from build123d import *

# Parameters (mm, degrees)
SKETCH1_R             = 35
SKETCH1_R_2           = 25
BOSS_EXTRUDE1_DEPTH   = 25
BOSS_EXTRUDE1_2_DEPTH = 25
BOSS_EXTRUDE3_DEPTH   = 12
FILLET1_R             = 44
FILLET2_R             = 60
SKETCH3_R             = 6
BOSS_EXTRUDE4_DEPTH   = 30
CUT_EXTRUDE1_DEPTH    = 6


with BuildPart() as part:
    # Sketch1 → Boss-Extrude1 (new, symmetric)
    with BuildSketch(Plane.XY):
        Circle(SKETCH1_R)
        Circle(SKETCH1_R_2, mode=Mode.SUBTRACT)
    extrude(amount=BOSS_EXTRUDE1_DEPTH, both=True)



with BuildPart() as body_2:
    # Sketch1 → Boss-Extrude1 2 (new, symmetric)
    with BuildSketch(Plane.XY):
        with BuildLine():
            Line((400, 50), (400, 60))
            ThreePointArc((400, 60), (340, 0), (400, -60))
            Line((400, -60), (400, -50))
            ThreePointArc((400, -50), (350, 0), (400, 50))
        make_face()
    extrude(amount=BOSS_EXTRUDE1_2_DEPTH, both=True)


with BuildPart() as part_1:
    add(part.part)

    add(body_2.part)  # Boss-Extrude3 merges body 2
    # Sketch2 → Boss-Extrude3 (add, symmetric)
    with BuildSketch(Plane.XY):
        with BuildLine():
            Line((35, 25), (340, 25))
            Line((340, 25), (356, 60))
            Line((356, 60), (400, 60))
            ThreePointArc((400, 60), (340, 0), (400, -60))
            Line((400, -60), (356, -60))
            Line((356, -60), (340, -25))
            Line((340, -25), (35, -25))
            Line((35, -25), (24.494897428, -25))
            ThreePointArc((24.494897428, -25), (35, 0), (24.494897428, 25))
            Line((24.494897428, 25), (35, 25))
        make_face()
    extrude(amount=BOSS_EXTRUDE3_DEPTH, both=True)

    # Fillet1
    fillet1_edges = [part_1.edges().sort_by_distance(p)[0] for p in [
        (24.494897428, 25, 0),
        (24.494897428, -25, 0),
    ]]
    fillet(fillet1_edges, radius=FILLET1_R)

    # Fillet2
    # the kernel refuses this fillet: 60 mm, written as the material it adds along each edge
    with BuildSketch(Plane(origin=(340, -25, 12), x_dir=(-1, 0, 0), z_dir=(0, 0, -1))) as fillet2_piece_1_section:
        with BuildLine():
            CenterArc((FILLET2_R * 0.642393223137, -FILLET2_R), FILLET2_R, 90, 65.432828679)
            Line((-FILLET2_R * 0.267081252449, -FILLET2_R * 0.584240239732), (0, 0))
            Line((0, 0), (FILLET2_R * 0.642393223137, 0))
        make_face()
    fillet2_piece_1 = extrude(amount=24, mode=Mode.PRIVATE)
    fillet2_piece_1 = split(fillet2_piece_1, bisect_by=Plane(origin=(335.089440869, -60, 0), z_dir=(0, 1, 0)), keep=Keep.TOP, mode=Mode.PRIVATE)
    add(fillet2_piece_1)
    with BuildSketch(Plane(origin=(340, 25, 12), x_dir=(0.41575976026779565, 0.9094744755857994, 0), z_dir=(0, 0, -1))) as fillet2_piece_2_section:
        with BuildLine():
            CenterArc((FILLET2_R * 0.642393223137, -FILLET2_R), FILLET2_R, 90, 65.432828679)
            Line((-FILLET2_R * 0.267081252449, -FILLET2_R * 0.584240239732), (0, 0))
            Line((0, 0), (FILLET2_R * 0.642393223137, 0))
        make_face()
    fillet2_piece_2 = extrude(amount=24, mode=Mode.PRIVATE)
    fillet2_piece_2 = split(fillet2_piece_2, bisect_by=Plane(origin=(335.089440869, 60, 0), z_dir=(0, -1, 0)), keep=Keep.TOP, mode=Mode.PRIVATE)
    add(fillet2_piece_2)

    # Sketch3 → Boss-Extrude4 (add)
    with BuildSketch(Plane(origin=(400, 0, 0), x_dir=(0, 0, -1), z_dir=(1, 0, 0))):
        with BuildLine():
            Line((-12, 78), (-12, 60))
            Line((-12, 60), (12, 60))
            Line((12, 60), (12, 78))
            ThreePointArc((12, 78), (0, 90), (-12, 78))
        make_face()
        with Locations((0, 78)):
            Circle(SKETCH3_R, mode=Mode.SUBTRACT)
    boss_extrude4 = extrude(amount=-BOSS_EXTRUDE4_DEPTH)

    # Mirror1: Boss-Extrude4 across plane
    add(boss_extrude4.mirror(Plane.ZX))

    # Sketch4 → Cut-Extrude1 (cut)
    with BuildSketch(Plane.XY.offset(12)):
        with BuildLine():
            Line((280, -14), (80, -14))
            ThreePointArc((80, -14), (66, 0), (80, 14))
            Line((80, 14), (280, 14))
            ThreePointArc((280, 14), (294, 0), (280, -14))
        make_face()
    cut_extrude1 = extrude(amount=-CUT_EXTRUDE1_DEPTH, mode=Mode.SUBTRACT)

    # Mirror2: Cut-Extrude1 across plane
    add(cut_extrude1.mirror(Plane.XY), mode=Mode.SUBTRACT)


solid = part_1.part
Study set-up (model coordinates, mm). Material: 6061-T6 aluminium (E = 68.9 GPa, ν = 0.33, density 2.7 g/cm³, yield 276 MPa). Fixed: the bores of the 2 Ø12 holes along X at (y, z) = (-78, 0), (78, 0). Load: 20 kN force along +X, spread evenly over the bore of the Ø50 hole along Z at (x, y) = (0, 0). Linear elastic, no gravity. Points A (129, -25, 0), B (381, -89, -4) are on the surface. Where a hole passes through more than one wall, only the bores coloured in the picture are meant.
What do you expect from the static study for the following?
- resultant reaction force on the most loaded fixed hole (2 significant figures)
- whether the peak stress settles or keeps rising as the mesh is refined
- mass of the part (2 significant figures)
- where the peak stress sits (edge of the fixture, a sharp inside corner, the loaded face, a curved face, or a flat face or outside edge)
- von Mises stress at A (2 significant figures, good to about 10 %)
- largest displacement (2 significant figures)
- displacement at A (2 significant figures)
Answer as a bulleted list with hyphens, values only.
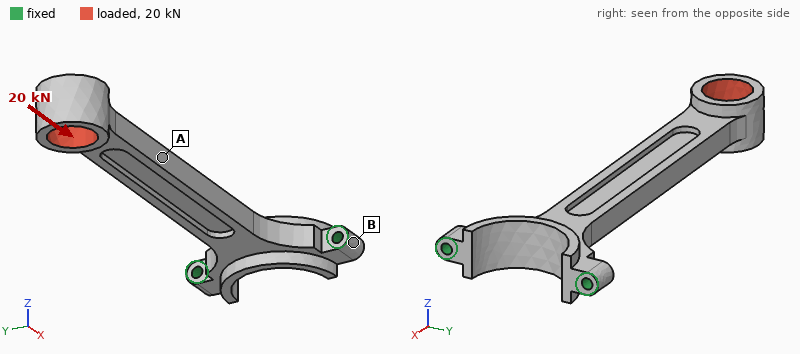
- 13 kN
- keeps rising
- 1.5 kg
- edge of the fixture
- 23 MPa
- 0.19 mm
- 0.10 mm
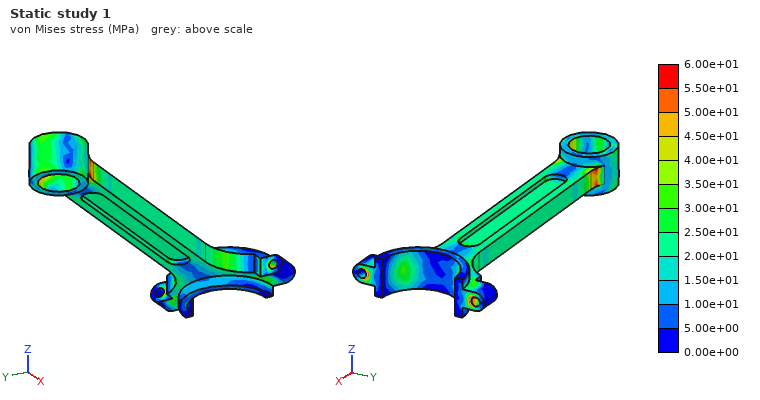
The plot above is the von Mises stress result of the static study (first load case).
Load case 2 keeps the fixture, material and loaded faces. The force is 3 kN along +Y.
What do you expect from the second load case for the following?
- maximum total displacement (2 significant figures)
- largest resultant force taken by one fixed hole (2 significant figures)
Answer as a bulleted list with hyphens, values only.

- 3.4 mm
- 11 kN
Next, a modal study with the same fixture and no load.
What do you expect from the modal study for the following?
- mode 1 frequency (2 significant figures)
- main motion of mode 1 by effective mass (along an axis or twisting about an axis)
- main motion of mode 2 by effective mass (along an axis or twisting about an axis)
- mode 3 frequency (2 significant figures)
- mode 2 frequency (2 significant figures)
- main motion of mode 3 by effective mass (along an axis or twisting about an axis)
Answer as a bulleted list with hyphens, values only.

- 92 Hz
- along Z
- along Y
- 570 Hz
- 250 Hz
- along Z
